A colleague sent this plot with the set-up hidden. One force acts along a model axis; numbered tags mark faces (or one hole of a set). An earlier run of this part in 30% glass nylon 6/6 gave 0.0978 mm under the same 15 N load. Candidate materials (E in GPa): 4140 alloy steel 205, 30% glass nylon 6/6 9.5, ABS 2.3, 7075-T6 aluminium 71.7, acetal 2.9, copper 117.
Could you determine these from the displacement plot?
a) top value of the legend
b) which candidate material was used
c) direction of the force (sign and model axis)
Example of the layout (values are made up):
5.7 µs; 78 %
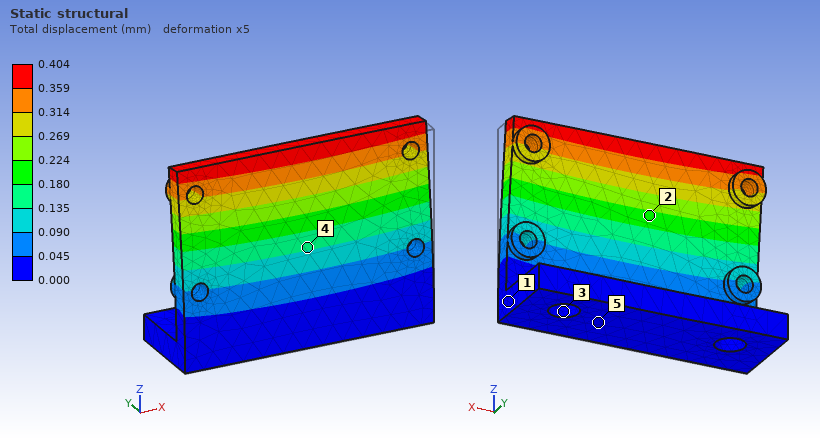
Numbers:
0.404 mm; ABS; +Y
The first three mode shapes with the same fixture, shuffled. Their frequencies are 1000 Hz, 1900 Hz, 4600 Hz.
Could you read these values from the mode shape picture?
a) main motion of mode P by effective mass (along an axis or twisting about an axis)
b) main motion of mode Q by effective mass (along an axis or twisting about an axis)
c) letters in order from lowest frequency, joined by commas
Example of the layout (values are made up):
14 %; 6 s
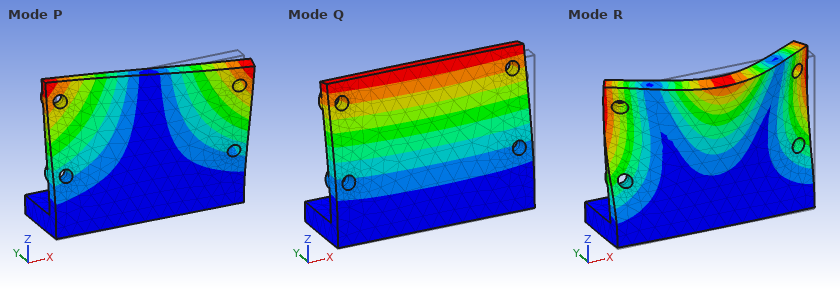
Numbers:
twisting about Z; along Y; Q, P, R
